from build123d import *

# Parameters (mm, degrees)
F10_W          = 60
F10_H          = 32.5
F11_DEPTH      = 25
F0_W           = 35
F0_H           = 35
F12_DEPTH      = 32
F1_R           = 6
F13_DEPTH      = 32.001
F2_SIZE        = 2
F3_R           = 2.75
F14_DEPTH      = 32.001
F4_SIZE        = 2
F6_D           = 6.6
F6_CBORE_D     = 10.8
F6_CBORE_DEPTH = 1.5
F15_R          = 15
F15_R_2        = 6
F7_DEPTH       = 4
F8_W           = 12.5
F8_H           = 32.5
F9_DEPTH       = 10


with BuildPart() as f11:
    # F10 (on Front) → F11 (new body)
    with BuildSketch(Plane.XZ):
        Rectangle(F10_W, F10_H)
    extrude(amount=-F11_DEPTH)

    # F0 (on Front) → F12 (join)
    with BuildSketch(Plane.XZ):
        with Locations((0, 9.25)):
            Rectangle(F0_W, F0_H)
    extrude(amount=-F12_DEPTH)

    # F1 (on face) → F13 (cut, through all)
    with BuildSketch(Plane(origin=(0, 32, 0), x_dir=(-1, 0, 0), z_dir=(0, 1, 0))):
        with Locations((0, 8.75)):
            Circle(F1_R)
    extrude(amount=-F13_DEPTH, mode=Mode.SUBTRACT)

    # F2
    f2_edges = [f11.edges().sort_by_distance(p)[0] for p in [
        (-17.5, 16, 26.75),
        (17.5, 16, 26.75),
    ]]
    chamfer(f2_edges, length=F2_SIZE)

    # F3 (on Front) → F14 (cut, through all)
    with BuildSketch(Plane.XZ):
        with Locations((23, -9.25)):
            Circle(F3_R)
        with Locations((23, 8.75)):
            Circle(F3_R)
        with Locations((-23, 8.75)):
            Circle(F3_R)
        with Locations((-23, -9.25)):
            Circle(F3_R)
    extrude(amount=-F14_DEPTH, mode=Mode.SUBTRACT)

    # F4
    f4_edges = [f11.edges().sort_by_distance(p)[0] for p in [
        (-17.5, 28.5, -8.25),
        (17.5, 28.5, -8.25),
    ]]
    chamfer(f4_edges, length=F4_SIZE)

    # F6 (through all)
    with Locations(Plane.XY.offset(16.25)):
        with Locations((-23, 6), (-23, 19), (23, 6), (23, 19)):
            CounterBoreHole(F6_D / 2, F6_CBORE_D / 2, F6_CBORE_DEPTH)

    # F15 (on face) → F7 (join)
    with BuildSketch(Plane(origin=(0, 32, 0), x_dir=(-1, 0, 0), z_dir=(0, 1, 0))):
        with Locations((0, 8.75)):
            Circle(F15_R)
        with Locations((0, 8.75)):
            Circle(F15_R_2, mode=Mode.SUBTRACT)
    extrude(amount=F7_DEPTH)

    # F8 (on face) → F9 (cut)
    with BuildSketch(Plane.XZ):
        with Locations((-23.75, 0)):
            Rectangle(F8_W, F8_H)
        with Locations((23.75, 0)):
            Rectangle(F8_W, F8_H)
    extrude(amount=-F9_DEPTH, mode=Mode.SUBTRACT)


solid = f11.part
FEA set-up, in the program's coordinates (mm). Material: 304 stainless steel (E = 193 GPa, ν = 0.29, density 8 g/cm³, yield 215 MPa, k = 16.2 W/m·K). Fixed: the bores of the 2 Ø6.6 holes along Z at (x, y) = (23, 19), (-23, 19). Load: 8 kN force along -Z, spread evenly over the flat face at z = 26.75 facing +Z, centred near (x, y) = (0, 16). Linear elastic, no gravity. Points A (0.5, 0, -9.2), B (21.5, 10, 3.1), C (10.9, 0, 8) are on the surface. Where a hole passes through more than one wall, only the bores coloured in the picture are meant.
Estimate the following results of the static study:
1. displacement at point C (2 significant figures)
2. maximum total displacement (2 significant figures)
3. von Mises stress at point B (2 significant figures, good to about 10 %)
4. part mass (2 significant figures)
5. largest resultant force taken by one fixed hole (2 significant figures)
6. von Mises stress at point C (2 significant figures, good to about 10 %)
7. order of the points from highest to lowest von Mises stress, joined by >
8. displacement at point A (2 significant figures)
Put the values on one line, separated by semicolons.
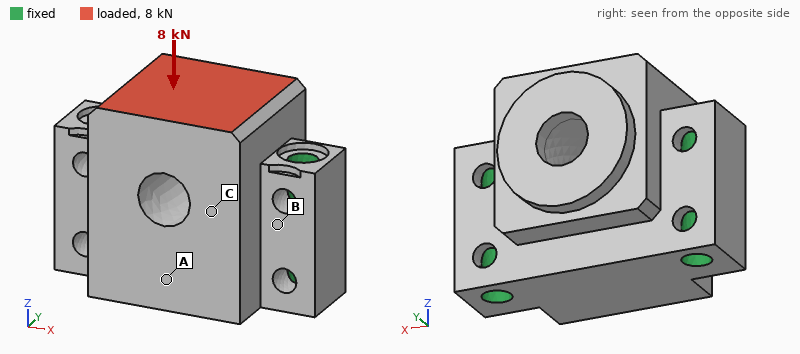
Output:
2.0 µm; 3.3 µm; 13 MPa; 430 g; 4.2 kN; 7.5 MPa; B > C > A; 1.7 µm
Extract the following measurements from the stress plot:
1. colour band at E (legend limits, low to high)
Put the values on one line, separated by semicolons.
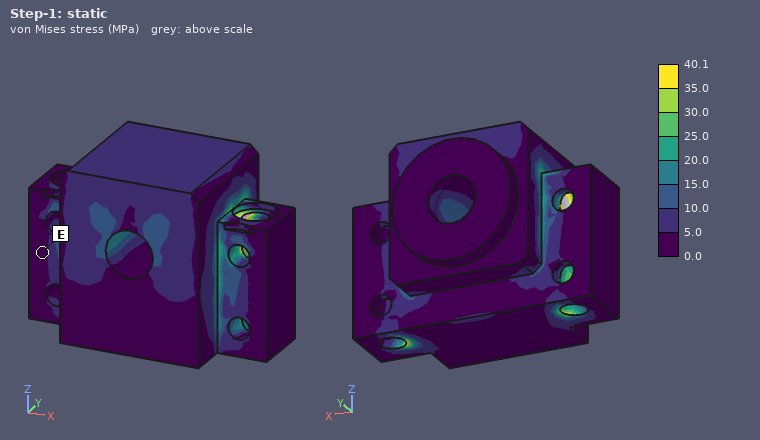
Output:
0.0 to 5.0 MPa
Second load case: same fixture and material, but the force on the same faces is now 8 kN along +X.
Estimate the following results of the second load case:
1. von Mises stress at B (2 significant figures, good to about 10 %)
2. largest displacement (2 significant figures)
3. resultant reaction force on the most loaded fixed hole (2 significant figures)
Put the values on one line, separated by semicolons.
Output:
14 MPa; 4.8 µm; 5.4 kN
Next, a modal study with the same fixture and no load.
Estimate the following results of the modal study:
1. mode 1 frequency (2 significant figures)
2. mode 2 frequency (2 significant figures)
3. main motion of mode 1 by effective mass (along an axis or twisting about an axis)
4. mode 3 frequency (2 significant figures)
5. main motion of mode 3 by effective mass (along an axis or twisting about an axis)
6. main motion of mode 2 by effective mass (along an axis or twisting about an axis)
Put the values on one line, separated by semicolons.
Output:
12 kHz; 21 kHz; along Y; 23 kHz; along Y; along Z
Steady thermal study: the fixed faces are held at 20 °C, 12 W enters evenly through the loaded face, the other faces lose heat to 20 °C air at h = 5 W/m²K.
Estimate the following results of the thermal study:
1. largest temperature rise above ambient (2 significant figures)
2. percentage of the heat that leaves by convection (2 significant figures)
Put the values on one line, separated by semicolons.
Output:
23 K; 3.0 %
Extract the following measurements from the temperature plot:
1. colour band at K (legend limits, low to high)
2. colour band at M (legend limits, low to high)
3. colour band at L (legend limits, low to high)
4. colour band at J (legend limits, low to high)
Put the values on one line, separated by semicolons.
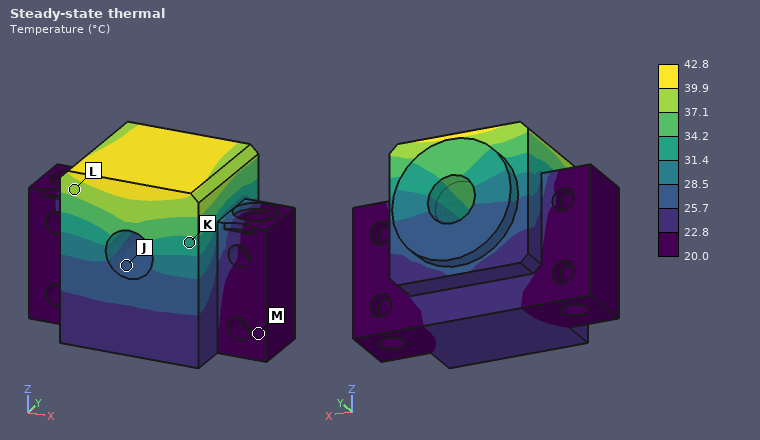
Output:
31.4 to 34.2 °C; 20.0 to 22.8 °C; 37.1 to 39.9 °C; 25.7 to 28.5 °C
